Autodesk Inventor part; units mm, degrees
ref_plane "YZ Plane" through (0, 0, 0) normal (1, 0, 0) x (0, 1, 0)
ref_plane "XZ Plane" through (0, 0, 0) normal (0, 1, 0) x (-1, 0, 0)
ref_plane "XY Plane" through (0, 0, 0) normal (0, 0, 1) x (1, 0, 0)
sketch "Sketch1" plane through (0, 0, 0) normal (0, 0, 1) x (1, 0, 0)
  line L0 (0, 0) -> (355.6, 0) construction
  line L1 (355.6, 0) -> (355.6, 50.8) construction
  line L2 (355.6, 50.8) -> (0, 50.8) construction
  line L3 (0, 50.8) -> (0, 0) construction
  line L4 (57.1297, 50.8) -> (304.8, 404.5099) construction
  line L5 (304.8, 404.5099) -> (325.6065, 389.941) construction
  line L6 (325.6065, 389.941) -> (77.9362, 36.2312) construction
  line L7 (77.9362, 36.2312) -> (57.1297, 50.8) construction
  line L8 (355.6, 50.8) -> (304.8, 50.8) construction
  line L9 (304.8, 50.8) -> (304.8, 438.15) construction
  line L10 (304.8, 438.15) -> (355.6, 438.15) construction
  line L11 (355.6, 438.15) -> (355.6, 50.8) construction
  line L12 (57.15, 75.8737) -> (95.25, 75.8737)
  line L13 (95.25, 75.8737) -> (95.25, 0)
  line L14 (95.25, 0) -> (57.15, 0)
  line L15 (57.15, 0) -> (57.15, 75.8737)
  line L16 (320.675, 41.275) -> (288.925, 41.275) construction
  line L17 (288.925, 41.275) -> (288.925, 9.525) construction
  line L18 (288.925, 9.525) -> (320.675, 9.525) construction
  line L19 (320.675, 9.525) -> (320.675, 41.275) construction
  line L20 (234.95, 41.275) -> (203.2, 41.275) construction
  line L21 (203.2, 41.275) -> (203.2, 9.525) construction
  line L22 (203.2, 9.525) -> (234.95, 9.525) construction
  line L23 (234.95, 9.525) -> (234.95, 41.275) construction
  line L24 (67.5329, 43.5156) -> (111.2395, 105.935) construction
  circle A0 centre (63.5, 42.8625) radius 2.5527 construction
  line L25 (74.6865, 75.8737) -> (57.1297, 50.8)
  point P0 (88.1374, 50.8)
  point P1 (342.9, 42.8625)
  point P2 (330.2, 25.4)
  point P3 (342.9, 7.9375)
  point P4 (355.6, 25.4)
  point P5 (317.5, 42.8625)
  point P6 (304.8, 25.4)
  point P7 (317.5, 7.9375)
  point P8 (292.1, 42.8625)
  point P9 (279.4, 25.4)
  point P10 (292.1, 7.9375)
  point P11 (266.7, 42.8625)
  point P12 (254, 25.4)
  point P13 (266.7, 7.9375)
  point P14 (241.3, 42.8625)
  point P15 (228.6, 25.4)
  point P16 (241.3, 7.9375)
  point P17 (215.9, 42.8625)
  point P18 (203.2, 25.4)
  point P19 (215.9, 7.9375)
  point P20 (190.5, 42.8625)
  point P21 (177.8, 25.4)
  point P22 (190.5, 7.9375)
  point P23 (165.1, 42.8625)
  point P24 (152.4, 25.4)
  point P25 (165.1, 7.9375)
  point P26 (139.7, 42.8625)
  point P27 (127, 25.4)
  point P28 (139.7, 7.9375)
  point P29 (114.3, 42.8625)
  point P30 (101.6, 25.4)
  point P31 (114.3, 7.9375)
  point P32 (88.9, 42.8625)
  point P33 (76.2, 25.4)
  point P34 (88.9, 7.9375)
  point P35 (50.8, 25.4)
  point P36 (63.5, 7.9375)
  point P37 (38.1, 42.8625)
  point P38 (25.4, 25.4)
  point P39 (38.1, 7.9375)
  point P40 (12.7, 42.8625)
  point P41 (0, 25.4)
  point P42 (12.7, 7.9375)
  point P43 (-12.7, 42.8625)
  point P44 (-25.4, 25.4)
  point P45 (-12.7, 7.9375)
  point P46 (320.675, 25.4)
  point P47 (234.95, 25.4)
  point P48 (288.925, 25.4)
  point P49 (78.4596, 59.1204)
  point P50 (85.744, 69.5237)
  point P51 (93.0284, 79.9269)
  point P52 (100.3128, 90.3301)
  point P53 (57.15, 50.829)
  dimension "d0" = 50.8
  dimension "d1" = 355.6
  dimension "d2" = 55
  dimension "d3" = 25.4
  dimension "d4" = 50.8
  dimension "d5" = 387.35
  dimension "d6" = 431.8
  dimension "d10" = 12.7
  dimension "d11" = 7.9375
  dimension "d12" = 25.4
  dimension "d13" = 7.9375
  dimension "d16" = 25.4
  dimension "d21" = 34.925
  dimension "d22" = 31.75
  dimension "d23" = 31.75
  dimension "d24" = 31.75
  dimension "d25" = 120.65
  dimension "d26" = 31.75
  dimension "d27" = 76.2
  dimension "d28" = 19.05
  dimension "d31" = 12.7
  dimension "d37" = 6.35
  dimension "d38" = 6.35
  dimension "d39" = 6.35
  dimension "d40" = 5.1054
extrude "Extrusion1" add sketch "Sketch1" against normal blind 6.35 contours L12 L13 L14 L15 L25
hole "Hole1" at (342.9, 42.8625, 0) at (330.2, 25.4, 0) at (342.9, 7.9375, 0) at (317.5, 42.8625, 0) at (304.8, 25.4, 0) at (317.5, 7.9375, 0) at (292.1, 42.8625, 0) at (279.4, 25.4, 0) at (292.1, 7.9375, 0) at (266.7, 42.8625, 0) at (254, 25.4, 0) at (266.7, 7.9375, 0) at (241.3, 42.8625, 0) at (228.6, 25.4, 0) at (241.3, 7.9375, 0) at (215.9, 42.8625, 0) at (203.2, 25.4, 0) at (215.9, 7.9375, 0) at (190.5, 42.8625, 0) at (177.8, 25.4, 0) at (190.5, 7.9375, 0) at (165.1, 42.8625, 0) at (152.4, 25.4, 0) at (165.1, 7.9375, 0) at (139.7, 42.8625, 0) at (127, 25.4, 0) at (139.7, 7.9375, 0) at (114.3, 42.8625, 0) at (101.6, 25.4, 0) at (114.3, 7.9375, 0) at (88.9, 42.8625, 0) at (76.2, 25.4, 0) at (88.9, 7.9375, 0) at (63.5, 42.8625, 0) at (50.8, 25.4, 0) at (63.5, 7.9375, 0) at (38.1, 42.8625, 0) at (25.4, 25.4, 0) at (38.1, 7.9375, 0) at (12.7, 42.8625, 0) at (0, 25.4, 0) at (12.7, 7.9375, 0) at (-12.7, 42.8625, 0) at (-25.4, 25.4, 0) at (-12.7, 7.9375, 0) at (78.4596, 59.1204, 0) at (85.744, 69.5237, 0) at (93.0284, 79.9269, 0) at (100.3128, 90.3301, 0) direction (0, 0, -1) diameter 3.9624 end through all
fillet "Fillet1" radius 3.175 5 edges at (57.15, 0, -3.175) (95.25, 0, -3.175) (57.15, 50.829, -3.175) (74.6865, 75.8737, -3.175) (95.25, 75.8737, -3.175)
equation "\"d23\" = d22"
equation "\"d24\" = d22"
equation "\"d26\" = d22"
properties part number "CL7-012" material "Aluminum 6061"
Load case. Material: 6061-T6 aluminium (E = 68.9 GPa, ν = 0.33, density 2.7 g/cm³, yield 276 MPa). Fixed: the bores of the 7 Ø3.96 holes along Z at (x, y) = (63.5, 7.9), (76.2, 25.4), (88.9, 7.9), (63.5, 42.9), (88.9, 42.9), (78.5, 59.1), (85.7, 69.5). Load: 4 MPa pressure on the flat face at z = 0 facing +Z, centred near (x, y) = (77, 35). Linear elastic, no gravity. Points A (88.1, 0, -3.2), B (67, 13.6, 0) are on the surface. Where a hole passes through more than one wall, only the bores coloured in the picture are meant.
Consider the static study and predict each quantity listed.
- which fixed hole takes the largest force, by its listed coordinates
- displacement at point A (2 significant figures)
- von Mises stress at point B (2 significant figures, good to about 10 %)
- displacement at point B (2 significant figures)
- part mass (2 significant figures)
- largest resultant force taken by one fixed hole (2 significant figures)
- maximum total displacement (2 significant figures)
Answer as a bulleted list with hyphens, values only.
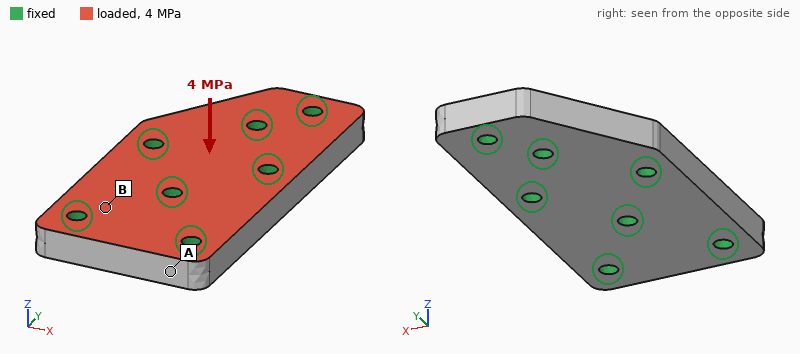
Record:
- (76.2, 25.4)
- 1.9 µm
- 18 MPa
- 3.4 µm
- 44 g
- 1.9 kN
- 11 µm
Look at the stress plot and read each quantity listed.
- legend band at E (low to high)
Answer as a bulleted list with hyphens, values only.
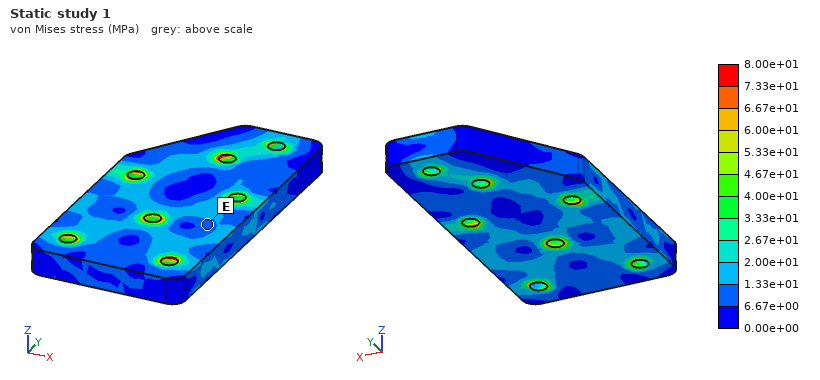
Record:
- 6.67e+00 to 1.33e+01 MPa
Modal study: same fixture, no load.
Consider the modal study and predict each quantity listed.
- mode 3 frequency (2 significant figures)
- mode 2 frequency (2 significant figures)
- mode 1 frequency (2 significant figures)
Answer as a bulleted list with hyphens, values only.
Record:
- 30 kHz
- 30 kHz
- 29 kHz
